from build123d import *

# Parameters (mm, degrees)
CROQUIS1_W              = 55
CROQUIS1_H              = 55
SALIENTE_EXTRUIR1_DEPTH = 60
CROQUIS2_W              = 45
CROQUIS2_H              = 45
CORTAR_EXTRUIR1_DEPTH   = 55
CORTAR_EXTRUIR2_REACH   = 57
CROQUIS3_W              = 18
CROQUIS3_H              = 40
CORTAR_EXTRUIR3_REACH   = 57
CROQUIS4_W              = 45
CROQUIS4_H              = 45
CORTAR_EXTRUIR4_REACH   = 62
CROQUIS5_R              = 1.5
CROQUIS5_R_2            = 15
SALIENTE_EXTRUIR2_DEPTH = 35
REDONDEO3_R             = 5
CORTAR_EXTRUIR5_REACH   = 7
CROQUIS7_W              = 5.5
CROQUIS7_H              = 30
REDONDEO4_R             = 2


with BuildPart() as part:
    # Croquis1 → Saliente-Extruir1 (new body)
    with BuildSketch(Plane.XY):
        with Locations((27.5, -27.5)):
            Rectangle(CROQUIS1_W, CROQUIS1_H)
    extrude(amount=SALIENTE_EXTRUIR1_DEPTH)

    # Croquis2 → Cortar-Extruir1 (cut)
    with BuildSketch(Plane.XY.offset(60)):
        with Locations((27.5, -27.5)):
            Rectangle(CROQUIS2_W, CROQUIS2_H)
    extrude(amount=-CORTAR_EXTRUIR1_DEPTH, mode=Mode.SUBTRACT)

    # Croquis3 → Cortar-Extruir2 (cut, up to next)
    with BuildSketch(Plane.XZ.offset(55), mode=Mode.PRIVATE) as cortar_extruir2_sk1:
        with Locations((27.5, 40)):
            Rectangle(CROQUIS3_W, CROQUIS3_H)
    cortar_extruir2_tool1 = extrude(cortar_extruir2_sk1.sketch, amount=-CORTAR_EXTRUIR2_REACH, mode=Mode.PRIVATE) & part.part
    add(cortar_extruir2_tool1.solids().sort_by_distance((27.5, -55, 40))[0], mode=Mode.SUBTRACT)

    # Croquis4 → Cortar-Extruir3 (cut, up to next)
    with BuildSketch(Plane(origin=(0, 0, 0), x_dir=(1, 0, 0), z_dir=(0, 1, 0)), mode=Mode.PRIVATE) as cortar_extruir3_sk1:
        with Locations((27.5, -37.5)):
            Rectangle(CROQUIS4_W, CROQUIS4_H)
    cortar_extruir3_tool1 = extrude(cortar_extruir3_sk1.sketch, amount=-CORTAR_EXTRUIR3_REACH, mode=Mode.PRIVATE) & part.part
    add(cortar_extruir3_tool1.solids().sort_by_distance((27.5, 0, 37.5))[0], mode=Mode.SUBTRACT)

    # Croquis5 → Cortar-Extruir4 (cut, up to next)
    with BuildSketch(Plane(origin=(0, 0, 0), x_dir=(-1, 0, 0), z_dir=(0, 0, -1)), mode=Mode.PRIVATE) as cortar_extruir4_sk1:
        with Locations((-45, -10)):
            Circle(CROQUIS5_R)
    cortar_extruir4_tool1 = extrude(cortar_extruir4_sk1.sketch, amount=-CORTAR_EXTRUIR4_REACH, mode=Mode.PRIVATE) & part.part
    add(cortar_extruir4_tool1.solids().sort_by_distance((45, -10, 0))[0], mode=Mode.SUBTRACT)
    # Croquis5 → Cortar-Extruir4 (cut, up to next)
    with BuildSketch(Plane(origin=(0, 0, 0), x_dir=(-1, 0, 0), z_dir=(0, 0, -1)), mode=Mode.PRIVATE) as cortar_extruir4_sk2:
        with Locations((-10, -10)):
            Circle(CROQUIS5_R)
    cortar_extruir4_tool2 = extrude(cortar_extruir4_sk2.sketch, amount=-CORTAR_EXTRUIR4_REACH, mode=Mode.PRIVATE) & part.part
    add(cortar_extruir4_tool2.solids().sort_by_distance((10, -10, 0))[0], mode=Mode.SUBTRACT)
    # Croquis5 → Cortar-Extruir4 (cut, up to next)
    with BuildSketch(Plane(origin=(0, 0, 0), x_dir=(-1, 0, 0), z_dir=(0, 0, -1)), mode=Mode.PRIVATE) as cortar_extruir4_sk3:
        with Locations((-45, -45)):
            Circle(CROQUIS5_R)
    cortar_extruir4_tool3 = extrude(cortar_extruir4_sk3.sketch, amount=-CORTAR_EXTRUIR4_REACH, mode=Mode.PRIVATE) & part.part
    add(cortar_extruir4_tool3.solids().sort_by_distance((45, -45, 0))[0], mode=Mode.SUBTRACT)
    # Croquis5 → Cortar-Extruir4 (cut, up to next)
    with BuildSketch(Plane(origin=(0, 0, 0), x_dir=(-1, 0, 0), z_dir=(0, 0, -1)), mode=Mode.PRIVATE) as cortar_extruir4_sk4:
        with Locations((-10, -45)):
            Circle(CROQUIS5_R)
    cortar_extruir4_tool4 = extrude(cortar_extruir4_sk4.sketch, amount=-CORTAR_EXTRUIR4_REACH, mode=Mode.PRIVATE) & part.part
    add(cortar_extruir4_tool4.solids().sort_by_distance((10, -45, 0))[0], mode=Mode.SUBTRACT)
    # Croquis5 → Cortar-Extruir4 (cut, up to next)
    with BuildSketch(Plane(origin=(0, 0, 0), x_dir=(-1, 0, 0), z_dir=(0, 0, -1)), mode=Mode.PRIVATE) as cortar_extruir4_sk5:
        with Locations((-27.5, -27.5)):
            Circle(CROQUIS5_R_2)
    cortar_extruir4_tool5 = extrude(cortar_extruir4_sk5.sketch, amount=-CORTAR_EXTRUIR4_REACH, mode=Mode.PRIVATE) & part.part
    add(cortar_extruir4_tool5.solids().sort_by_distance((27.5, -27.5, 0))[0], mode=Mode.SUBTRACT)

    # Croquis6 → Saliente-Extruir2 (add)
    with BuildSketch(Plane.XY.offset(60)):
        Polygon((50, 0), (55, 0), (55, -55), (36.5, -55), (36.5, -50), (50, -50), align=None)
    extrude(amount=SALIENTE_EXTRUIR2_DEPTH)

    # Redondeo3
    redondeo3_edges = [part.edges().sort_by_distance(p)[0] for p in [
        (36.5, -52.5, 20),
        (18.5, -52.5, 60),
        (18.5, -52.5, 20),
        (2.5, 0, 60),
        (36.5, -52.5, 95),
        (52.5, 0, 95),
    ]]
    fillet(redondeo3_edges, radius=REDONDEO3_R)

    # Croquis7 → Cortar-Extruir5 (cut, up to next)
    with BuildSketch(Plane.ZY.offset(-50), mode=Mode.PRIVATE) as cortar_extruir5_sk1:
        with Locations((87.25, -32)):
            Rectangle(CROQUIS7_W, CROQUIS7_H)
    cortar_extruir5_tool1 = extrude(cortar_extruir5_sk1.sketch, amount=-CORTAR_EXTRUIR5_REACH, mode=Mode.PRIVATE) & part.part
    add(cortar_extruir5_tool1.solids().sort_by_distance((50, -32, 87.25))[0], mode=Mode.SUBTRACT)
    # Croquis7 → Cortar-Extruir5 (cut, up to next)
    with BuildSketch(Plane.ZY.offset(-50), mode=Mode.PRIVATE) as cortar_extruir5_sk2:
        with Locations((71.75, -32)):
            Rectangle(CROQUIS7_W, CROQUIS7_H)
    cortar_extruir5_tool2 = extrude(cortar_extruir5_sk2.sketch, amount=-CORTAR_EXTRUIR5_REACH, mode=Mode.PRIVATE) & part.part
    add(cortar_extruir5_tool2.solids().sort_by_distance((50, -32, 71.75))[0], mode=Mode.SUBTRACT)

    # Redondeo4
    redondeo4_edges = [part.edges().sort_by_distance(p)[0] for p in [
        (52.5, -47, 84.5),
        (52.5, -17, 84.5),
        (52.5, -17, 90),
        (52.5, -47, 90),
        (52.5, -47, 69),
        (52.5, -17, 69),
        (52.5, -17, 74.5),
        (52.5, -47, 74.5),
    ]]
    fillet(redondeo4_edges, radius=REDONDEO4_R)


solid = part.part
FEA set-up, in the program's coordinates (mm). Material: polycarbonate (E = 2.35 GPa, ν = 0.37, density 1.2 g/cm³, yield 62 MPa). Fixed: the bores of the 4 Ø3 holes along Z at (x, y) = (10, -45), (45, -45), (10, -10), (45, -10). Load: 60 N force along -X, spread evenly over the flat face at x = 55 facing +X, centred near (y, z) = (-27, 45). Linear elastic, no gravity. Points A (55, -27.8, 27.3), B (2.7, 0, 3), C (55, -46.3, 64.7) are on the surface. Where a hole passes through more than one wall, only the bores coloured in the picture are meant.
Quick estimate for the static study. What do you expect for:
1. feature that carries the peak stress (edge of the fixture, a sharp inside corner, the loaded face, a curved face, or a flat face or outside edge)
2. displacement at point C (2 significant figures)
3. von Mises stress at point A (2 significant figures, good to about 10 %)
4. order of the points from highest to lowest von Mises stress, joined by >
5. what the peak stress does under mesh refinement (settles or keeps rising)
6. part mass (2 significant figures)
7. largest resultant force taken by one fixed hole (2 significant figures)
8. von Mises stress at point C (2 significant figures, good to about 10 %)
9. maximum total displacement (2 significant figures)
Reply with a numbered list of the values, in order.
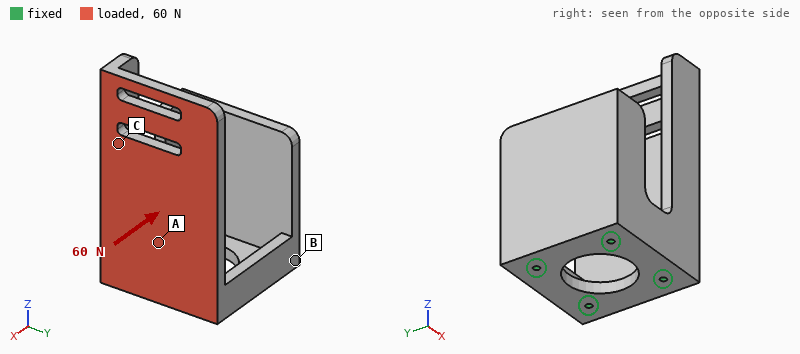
1. edge of the fixture
2. 0.33 mm
3. 1.8 MPa
4. A > C > B
5. keeps rising
6. 76 g
7. 60 N
8. 1.1 MPa
9. 1.2 mm
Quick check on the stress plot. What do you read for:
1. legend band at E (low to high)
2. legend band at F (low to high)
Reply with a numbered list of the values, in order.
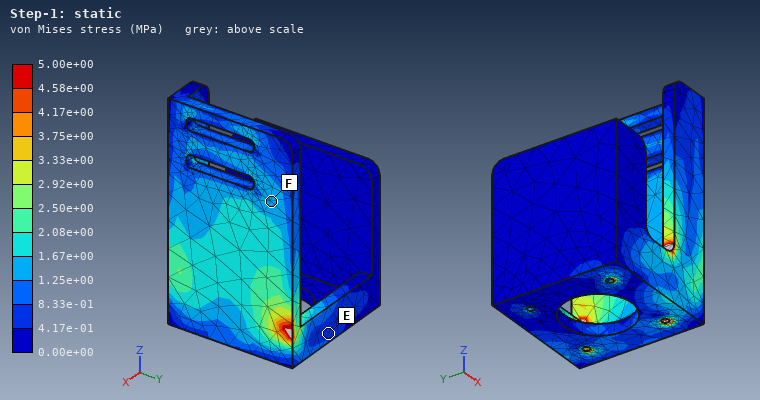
1. 4.17e-01 to 8.33e-01 MPa
2. 1.25e+00 to 1.67e+00 MPa
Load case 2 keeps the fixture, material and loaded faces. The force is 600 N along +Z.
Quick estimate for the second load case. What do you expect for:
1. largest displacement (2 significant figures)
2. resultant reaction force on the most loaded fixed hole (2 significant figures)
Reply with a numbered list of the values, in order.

1. 1.5 mm
2. 380 N
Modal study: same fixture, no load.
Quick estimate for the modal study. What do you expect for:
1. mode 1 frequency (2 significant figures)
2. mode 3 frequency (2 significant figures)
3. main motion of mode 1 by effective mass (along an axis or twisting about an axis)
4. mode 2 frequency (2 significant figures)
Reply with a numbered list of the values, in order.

1. 280 Hz
2. 590 Hz
3. along X
4. 530 Hz
